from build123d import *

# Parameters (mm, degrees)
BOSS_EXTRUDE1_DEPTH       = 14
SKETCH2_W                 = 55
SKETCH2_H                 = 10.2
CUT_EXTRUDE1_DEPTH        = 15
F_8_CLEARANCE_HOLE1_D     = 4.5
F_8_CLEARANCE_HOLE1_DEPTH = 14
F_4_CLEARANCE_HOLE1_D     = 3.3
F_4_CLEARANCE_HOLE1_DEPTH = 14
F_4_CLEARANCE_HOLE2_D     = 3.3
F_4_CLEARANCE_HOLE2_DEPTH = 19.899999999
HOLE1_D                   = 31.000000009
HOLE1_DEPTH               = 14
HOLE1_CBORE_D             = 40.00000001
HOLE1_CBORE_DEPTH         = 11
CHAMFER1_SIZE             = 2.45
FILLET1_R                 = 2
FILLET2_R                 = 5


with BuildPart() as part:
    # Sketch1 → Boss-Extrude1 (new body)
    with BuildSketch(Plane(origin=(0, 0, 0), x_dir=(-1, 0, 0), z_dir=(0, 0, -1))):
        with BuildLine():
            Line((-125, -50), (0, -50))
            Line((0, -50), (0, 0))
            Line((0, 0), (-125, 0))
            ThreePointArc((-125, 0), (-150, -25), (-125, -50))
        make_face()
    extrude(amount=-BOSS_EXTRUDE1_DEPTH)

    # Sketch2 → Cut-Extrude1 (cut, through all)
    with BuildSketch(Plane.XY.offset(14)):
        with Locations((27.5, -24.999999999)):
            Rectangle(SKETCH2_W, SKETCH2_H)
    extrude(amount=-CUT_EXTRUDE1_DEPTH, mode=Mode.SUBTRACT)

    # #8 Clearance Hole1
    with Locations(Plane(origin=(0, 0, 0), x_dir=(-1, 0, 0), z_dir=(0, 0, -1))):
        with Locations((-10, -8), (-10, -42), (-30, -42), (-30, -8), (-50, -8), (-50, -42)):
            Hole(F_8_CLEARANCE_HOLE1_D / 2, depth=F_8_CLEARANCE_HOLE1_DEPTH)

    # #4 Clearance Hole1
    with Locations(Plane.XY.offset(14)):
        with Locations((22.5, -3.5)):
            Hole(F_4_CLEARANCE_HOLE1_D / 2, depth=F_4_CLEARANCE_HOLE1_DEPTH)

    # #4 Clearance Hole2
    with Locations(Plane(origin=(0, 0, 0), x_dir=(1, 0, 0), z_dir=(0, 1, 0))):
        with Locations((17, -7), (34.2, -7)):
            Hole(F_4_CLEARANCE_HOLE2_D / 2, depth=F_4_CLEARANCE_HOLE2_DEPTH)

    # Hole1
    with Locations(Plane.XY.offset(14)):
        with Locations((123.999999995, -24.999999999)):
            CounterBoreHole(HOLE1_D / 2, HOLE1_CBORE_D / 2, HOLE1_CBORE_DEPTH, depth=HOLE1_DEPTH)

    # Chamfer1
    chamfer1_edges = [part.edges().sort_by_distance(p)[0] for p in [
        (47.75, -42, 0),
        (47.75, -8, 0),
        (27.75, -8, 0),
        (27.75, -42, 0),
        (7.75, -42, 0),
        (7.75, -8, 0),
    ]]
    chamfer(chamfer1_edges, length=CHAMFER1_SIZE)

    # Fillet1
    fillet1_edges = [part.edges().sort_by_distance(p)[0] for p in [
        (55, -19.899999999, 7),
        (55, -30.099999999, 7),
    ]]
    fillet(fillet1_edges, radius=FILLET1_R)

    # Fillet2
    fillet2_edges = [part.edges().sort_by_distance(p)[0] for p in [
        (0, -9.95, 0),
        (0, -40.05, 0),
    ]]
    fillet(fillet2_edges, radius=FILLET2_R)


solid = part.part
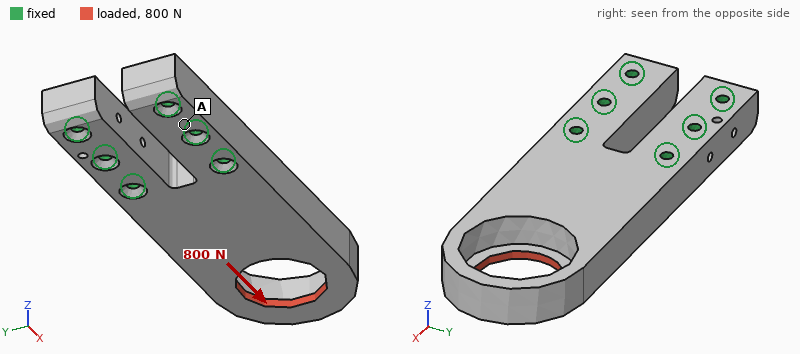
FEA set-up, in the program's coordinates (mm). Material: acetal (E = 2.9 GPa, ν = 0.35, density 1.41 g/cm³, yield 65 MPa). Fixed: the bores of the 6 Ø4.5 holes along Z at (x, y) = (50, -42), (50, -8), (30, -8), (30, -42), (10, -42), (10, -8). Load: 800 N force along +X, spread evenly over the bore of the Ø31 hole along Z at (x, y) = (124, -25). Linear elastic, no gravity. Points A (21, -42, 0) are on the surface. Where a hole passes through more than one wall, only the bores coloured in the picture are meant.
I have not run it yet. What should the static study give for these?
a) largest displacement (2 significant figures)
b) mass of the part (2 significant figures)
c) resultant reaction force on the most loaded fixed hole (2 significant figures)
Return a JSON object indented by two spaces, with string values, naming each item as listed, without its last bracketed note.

{
  "largest displacement": "0.86 mm",
  "mass of the part": "110 g",
  "resultant reaction force on the most loaded fixed hole": "320 N"
}
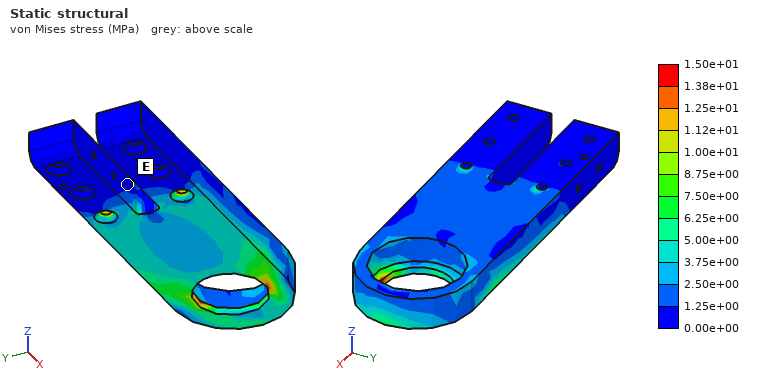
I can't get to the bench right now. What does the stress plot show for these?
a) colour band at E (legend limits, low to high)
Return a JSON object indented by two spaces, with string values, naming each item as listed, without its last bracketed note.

{
  "colour band at E": "0.00e+00 to 1.25e+00 MPa"
}
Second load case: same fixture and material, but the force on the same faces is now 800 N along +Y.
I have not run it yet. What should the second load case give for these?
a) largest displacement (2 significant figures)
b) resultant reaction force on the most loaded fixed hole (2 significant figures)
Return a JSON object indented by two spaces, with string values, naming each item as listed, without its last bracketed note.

{
  "largest displacement": "0.97 mm",
  "resultant reaction force on the most loaded fixed hole": "1.5 kN"
}
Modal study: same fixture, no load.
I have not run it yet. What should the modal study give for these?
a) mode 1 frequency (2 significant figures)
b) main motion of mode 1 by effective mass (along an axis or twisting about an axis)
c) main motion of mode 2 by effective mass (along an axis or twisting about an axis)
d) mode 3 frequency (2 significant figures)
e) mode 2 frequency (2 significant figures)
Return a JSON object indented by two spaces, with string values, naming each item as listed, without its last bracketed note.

{
  "mode 1 frequency": "430 Hz",
  "main motion of mode 1 by effective mass": "along Z",
  "main motion of mode 2 by effective mass": "along Y",
  "mode 3 frequency": "1300 Hz",
  "mode 2 frequency": "1100 Hz"
}
